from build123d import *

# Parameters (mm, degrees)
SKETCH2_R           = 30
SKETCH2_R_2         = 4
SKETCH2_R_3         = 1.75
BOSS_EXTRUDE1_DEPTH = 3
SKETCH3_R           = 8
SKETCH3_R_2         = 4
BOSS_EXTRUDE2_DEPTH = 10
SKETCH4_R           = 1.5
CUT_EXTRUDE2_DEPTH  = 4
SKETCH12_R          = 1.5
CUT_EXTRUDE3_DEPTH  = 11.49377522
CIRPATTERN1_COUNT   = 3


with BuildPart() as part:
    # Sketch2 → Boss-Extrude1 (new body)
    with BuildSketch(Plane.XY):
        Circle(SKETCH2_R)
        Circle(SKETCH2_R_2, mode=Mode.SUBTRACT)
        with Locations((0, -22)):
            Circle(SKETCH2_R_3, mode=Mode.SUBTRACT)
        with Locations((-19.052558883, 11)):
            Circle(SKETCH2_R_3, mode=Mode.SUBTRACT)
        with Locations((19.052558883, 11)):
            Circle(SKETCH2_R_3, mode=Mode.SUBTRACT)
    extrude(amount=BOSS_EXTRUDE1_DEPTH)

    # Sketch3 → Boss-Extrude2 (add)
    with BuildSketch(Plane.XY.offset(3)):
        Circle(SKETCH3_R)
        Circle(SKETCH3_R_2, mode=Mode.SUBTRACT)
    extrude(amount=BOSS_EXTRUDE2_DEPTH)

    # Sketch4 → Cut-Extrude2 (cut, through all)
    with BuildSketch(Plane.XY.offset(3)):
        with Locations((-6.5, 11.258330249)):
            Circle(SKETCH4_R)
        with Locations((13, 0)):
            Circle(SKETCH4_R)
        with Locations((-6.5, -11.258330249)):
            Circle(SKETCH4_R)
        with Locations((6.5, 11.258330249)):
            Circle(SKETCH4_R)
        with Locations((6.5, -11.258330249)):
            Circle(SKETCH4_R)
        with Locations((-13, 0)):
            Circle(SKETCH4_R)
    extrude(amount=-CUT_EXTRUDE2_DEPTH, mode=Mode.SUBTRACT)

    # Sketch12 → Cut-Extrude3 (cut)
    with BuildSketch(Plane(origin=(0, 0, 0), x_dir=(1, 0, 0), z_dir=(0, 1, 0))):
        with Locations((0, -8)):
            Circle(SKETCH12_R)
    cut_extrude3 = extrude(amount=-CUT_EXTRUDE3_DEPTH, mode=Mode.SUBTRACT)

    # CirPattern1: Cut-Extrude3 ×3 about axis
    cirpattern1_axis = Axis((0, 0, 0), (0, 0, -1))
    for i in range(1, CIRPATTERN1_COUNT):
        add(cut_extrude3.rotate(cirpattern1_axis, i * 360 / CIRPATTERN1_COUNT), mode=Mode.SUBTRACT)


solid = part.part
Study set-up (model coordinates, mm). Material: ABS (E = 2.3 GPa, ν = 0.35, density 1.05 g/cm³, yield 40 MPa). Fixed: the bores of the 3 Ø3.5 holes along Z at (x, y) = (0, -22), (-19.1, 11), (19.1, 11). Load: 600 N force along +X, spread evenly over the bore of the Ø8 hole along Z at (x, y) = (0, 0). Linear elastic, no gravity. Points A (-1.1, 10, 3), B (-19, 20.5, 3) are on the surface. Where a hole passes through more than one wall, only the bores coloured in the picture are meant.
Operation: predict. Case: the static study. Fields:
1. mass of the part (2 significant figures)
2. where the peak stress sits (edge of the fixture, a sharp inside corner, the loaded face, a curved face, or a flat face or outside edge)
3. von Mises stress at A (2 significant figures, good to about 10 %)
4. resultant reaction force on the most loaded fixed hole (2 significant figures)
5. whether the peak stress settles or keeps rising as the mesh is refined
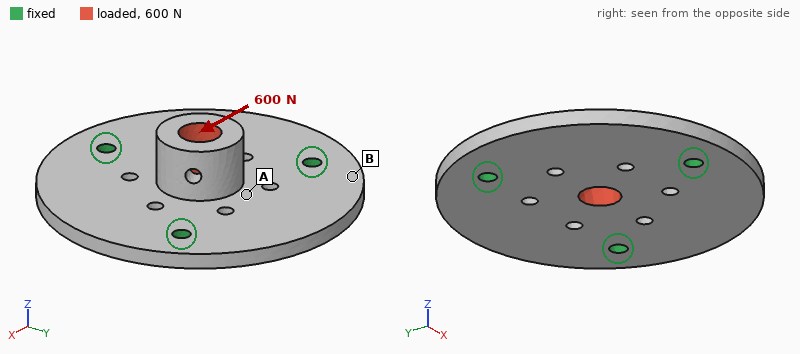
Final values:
10 g
edge of the fixture
12 MPa
230 N
keeps rising
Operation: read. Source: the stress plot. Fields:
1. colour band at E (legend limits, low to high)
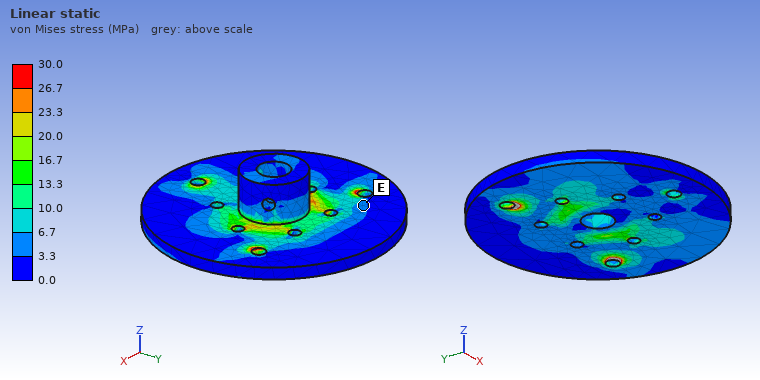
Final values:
3.3 to 6.7 MPa
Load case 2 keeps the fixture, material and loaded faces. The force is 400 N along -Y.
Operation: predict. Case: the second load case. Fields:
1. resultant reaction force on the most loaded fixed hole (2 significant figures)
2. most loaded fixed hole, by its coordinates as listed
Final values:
170 N
(0, -22)
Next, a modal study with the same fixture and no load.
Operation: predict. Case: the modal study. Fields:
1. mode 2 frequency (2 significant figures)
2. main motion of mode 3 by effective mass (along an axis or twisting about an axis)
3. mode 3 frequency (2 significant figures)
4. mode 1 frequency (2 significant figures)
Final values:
1800 Hz
along Z
2000 Hz
1800 Hz
